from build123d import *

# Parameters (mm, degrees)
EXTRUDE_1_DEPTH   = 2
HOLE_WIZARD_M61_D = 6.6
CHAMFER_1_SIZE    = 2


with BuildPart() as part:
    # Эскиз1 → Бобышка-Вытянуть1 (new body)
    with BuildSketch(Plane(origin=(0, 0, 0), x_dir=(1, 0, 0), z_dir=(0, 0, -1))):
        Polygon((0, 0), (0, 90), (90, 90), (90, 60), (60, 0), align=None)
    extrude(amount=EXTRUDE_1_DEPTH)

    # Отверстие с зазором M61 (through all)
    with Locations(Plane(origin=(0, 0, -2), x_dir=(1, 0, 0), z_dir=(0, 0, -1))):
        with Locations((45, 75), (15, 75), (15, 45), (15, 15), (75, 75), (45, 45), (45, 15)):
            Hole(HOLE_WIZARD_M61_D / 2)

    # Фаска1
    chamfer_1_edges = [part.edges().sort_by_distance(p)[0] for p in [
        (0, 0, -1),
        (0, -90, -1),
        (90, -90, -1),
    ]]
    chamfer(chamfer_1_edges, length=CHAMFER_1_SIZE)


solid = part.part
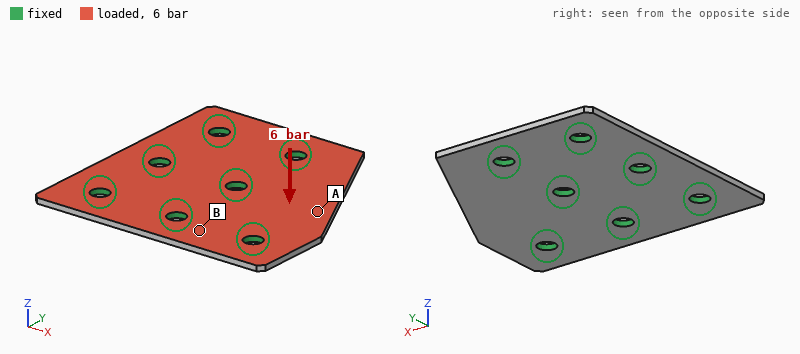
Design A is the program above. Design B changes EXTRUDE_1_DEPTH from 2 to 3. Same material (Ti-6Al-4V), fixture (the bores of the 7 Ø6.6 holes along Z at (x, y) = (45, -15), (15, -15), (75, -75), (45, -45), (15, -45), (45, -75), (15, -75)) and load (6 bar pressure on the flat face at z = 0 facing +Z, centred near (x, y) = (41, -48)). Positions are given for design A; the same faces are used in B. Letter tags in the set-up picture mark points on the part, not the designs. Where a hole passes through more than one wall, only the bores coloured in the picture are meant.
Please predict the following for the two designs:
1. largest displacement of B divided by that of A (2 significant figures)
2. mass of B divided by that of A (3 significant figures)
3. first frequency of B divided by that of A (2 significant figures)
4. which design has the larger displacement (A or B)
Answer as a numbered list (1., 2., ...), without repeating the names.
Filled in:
1. 0.31
2. 1.50
3. 1.5
4. A
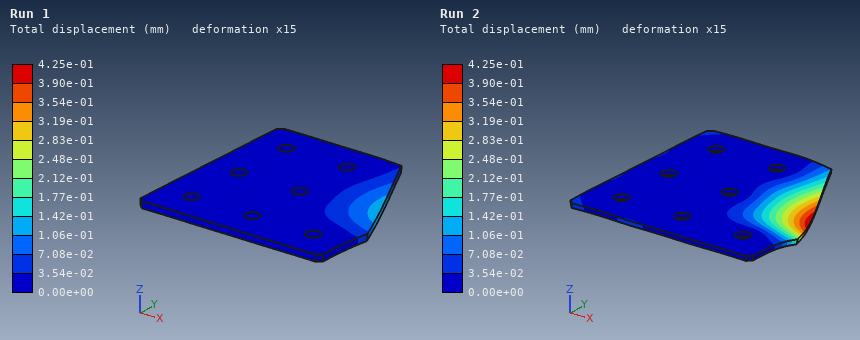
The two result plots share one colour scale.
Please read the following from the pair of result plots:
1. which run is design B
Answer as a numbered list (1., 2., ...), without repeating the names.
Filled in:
1. Run 1
